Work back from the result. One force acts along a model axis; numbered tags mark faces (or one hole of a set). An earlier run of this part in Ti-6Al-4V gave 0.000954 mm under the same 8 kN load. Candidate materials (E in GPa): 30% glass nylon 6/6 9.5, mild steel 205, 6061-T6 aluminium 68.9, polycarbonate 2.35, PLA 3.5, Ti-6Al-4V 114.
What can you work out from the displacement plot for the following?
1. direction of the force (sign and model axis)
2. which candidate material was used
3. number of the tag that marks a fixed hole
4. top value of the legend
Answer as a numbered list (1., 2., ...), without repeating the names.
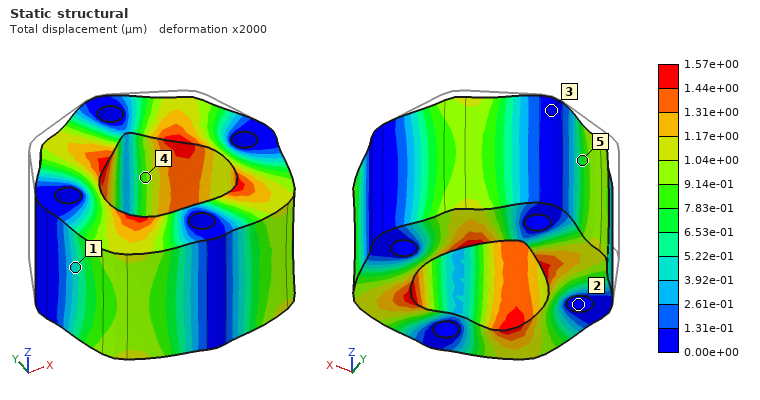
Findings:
1. -Y
2. 6061-T6 aluminium
3. 2
4. 1.57e+00 µm
